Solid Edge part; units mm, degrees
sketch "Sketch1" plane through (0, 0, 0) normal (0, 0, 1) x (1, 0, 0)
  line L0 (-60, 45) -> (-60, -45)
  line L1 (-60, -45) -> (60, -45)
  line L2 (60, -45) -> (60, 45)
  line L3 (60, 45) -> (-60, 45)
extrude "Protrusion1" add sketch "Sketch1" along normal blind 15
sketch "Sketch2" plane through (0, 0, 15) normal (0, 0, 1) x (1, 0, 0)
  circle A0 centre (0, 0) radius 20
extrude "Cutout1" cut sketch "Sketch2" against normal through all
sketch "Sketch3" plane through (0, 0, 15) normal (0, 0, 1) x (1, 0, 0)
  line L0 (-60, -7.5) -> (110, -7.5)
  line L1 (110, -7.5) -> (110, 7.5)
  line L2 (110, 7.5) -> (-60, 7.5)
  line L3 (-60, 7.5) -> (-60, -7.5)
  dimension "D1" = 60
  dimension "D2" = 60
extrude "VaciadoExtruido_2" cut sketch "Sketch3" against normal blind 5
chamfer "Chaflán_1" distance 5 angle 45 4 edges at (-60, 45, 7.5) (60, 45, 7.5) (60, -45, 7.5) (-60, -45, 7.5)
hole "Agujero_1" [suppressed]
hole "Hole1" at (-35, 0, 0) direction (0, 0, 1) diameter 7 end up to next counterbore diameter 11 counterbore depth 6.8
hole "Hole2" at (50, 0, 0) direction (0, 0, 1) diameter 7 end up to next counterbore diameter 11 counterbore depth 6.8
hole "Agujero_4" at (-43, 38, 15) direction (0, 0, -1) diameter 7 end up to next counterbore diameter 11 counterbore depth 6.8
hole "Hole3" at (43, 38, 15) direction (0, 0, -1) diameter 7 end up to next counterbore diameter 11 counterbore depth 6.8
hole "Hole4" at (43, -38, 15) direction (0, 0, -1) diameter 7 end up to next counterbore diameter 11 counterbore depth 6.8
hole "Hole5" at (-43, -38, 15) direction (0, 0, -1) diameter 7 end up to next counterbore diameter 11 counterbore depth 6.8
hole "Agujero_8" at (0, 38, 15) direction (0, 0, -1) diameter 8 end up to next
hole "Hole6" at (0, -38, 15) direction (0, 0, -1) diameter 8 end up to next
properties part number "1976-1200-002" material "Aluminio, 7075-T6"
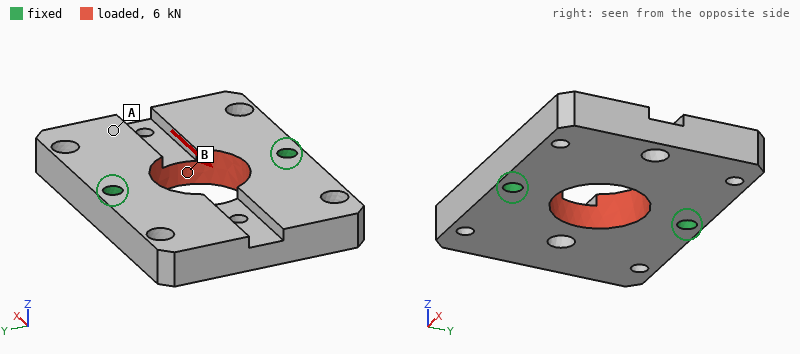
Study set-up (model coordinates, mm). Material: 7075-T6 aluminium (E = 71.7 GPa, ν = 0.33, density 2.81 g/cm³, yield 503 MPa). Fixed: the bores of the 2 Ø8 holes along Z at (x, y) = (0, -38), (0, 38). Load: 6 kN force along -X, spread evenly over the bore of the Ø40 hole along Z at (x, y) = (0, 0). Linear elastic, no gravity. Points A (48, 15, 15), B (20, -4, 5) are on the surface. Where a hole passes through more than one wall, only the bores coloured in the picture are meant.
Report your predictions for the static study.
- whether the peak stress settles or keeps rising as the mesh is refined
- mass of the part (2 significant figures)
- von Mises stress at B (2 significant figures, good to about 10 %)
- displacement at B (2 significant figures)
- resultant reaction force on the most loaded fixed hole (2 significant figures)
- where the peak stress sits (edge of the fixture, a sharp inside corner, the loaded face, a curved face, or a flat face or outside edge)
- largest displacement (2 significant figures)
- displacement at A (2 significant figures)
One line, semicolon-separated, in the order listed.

keeps rising; 360 g; 3.5 MPa; 4.1 µm; 3.0 kN; edge of the fixture; 4.6 µm; 3.4 µm
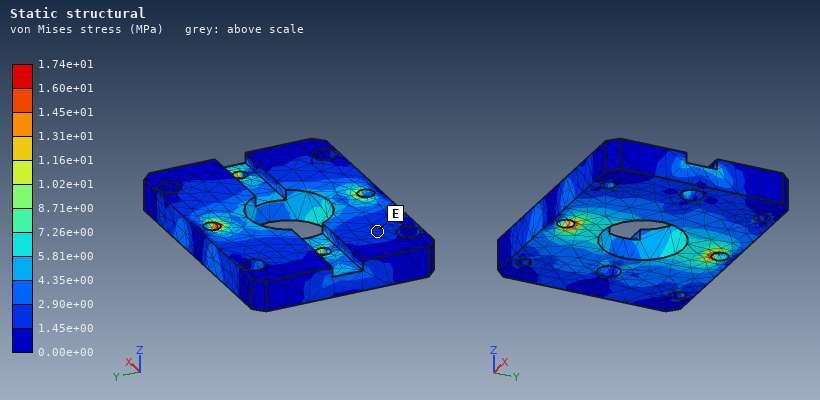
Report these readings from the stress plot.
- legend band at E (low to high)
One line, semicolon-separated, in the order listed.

1.45e+00 to 2.90e+00 MPa
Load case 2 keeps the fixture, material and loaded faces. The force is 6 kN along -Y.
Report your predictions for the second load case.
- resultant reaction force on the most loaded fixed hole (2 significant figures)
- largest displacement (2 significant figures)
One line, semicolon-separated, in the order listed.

3.0 kN; 4.1 µm
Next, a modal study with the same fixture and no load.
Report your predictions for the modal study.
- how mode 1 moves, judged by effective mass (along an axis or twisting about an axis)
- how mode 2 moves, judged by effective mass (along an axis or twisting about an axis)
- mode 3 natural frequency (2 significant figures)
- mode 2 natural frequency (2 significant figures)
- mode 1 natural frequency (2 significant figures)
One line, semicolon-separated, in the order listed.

twisting about Y; along Z; 5000 Hz; 2800 Hz; 2400 Hz
